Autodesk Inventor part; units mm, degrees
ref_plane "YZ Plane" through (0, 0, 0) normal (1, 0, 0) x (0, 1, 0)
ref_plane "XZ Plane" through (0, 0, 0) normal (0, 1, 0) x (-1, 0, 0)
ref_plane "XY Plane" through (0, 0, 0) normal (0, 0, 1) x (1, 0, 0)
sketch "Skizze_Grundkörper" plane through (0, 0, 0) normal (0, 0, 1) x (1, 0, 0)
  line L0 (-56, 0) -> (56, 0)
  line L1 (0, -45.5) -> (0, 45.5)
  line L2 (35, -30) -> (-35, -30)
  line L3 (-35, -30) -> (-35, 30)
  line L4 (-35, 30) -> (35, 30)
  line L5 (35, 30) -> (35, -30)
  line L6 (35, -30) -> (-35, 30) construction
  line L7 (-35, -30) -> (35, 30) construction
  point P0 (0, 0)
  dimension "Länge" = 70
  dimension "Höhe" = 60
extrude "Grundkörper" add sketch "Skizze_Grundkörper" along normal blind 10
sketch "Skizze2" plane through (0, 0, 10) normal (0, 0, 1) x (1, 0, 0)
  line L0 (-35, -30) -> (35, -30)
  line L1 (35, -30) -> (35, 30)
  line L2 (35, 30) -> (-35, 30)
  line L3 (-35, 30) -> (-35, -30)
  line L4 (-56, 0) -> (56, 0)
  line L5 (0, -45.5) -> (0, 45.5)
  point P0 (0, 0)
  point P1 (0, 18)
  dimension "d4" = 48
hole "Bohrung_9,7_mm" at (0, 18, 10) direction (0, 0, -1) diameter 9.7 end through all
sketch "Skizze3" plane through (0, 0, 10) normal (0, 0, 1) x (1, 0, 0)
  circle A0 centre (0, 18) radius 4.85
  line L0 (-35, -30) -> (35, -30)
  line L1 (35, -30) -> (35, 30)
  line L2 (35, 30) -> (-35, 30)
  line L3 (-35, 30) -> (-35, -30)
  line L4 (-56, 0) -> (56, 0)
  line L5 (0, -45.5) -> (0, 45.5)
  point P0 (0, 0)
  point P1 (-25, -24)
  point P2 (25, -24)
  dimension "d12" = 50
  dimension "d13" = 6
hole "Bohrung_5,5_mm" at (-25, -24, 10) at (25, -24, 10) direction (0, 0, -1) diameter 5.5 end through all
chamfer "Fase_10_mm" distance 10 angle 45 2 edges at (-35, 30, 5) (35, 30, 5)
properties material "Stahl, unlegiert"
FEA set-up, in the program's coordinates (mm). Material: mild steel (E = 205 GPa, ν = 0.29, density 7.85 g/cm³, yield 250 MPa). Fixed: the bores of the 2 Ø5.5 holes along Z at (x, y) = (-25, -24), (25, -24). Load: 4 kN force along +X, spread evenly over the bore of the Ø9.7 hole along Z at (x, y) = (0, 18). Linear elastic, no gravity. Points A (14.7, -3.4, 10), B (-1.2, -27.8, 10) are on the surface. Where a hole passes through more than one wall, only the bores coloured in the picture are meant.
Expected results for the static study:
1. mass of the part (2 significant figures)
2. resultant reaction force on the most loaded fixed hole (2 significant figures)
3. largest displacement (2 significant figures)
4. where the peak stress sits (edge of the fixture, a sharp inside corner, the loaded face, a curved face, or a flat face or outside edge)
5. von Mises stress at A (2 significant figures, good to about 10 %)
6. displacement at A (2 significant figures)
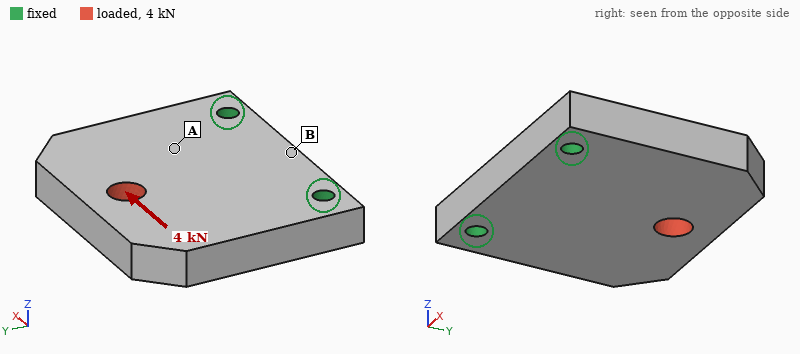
310 g
3.7 kN
7.5 µm
edge of the fixture
14 MPa
2.8 µm
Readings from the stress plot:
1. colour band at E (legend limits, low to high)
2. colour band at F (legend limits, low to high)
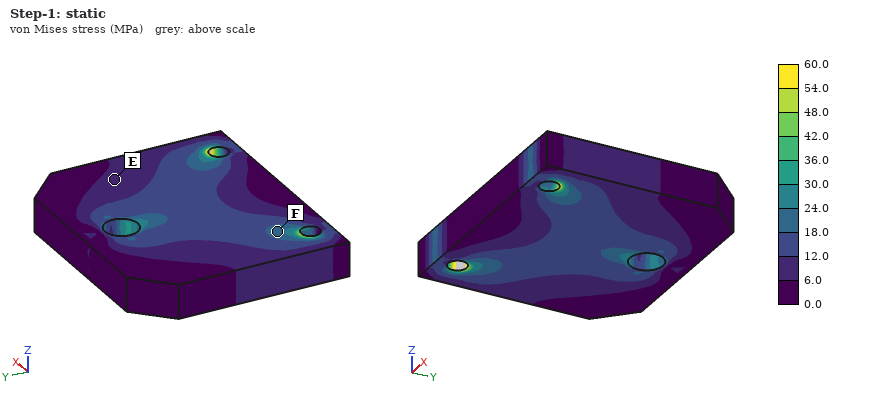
6.0 to 12.0 MPa
18.0 to 24.0 MPa
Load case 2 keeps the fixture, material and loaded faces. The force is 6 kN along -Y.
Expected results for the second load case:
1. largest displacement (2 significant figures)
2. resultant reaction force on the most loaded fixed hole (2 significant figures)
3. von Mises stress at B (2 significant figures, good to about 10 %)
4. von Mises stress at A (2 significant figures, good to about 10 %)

5.2 µm
3.1 kN
5.8 MPa
14 MPa
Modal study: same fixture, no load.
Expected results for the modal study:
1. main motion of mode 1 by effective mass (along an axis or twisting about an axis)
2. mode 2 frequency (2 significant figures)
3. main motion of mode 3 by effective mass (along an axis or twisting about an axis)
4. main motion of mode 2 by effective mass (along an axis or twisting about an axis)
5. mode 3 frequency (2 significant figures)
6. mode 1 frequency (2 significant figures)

along Z
5700 Hz
along X
twisting about Y
10 kHz
2500 Hz
